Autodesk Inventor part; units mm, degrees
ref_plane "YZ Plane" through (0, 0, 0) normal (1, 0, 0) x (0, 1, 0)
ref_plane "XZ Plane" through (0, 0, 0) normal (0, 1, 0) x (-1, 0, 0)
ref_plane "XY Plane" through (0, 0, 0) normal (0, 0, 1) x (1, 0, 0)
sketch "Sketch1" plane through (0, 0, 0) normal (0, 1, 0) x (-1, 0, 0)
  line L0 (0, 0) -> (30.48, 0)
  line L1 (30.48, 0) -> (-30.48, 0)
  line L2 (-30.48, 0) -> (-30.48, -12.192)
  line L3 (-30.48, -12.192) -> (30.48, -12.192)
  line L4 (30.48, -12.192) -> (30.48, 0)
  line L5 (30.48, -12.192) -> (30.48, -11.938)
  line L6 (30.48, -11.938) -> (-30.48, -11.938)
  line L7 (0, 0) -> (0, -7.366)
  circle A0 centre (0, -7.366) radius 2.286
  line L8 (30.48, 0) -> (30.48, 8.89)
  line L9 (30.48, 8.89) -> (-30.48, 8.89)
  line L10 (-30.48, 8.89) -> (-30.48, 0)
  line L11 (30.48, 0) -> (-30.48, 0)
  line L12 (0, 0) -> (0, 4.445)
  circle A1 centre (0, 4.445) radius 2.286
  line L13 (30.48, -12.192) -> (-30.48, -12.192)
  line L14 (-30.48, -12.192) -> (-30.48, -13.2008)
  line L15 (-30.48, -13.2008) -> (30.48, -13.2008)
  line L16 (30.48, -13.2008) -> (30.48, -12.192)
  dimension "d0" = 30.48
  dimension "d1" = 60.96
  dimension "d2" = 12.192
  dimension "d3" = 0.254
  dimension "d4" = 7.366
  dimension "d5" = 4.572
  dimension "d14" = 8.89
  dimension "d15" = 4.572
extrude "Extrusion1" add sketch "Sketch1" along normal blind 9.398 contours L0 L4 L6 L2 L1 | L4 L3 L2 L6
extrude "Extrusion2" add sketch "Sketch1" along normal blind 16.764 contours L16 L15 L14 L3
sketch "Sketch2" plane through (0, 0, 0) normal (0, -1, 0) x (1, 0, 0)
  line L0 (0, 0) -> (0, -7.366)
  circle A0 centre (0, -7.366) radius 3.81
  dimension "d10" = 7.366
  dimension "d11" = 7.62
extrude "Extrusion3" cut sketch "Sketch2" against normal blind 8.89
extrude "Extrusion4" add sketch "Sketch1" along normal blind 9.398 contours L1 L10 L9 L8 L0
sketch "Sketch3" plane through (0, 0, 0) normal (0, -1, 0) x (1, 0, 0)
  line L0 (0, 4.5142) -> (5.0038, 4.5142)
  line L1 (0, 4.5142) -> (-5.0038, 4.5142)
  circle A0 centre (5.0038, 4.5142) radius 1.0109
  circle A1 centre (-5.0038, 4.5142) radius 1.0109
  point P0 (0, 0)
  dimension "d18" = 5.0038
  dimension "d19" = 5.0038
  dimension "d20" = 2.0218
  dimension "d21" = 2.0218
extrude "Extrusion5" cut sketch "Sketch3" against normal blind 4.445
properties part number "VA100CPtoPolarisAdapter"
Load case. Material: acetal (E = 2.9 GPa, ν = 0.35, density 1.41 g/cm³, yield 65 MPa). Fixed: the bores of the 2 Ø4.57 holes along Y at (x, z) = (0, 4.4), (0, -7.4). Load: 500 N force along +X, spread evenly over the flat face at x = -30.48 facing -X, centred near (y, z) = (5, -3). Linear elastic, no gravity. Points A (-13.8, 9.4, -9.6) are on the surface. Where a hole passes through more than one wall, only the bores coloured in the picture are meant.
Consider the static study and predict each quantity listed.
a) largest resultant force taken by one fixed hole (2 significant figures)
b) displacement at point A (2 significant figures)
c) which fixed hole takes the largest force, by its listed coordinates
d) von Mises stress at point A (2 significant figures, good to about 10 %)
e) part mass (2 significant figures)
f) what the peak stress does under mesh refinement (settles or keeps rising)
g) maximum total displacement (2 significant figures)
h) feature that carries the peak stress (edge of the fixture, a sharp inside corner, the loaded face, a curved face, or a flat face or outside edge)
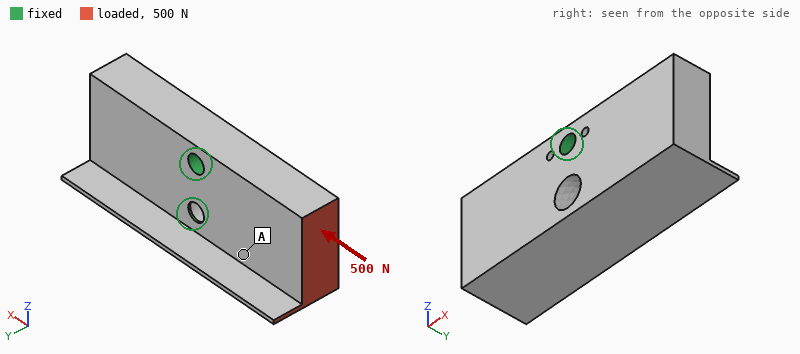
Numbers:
320 N
0.058 mm
(0, 4.4)
2.6 MPa
18 g
keeps rising
0.12 mm
edge of the fixture
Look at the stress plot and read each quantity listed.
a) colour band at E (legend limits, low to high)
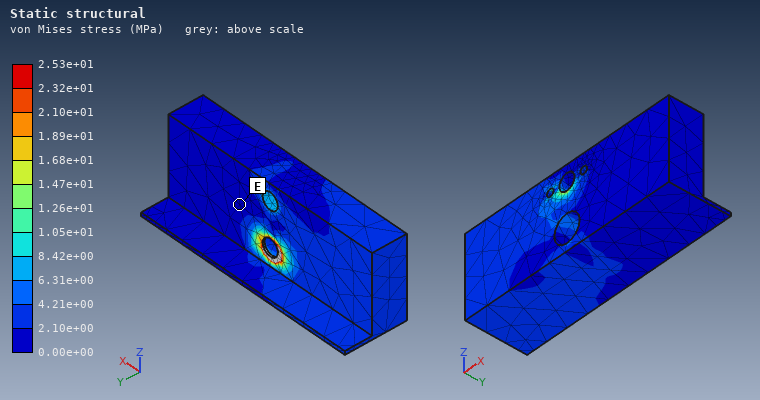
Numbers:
0.00e+00 to 2.10e+00 MPa
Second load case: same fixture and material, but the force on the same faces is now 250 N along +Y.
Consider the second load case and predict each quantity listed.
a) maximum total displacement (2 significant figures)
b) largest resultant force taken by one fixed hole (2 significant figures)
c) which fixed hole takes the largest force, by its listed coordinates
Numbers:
0.76 mm
260 N
(0, 4.4)
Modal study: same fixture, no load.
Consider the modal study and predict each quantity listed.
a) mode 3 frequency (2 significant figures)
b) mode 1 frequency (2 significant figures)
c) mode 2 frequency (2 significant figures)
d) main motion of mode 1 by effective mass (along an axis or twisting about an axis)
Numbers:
2300 Hz
1600 Hz
2200 Hz
twisting about Z
